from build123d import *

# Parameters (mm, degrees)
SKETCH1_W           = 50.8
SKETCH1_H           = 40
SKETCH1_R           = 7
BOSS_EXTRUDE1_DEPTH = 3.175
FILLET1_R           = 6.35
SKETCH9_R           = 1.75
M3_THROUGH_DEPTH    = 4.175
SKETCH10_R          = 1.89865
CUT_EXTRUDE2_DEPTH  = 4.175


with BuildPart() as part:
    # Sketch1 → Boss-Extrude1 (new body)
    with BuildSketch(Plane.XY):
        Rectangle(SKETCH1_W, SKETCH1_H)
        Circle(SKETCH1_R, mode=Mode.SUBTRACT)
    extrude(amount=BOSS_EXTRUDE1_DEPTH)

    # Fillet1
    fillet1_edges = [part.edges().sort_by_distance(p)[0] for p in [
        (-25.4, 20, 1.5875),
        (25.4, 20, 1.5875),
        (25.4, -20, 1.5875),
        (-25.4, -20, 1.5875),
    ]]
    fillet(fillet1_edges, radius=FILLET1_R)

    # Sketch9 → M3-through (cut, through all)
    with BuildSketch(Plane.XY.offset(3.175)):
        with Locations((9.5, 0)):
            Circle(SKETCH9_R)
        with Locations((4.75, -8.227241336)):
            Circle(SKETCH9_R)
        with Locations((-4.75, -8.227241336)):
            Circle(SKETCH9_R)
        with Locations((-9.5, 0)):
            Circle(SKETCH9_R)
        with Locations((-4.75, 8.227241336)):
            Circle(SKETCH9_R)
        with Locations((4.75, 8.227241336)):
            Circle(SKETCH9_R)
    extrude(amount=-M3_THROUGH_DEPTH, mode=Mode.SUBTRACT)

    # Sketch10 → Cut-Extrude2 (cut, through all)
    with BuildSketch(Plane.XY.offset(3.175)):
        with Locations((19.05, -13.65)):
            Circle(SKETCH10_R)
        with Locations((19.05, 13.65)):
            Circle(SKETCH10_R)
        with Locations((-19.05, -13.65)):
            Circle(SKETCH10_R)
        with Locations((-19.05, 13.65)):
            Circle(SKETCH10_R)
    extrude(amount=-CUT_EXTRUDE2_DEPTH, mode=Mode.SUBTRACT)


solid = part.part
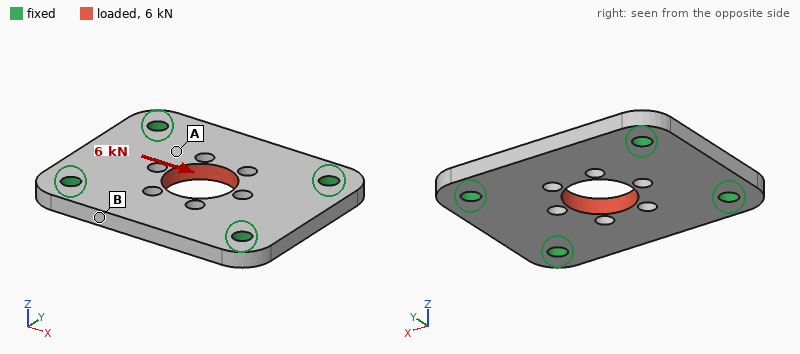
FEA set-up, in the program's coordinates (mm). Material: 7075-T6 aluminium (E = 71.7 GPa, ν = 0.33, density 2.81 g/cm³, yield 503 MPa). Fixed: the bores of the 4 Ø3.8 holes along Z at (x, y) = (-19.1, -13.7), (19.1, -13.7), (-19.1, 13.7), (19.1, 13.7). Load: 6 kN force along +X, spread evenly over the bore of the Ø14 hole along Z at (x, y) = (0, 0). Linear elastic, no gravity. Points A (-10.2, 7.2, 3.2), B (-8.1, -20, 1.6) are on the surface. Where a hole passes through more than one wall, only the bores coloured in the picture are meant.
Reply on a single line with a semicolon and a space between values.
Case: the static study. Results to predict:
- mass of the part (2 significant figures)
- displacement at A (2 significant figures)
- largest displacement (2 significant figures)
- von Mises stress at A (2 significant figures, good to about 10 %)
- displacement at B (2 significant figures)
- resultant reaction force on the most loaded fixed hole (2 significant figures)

16 g; 7.3 µm; 19 µm; 46 MPa; 3.2 µm; 1.6 kN
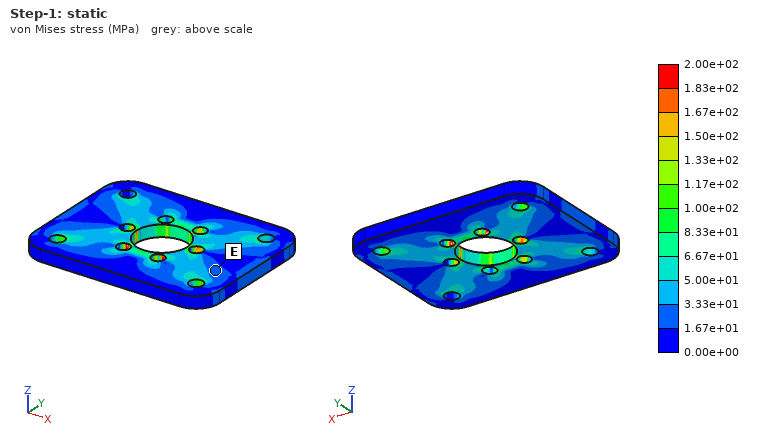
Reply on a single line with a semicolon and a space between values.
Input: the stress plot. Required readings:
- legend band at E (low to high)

1.67e+01 to 3.33e+01 MPa
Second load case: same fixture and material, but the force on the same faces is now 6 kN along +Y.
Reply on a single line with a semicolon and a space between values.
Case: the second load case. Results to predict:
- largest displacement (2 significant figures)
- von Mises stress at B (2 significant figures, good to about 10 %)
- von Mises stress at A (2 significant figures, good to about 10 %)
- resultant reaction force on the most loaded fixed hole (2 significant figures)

27 µm; 25 MPa; 61 MPa; 1.7 kN
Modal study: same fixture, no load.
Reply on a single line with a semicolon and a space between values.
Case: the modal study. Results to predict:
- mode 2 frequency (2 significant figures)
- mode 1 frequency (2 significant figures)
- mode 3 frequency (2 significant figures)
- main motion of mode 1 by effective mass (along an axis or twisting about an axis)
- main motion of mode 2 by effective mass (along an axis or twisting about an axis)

13 kHz; 11 kHz; 17 kHz; along Z; twisting about X
